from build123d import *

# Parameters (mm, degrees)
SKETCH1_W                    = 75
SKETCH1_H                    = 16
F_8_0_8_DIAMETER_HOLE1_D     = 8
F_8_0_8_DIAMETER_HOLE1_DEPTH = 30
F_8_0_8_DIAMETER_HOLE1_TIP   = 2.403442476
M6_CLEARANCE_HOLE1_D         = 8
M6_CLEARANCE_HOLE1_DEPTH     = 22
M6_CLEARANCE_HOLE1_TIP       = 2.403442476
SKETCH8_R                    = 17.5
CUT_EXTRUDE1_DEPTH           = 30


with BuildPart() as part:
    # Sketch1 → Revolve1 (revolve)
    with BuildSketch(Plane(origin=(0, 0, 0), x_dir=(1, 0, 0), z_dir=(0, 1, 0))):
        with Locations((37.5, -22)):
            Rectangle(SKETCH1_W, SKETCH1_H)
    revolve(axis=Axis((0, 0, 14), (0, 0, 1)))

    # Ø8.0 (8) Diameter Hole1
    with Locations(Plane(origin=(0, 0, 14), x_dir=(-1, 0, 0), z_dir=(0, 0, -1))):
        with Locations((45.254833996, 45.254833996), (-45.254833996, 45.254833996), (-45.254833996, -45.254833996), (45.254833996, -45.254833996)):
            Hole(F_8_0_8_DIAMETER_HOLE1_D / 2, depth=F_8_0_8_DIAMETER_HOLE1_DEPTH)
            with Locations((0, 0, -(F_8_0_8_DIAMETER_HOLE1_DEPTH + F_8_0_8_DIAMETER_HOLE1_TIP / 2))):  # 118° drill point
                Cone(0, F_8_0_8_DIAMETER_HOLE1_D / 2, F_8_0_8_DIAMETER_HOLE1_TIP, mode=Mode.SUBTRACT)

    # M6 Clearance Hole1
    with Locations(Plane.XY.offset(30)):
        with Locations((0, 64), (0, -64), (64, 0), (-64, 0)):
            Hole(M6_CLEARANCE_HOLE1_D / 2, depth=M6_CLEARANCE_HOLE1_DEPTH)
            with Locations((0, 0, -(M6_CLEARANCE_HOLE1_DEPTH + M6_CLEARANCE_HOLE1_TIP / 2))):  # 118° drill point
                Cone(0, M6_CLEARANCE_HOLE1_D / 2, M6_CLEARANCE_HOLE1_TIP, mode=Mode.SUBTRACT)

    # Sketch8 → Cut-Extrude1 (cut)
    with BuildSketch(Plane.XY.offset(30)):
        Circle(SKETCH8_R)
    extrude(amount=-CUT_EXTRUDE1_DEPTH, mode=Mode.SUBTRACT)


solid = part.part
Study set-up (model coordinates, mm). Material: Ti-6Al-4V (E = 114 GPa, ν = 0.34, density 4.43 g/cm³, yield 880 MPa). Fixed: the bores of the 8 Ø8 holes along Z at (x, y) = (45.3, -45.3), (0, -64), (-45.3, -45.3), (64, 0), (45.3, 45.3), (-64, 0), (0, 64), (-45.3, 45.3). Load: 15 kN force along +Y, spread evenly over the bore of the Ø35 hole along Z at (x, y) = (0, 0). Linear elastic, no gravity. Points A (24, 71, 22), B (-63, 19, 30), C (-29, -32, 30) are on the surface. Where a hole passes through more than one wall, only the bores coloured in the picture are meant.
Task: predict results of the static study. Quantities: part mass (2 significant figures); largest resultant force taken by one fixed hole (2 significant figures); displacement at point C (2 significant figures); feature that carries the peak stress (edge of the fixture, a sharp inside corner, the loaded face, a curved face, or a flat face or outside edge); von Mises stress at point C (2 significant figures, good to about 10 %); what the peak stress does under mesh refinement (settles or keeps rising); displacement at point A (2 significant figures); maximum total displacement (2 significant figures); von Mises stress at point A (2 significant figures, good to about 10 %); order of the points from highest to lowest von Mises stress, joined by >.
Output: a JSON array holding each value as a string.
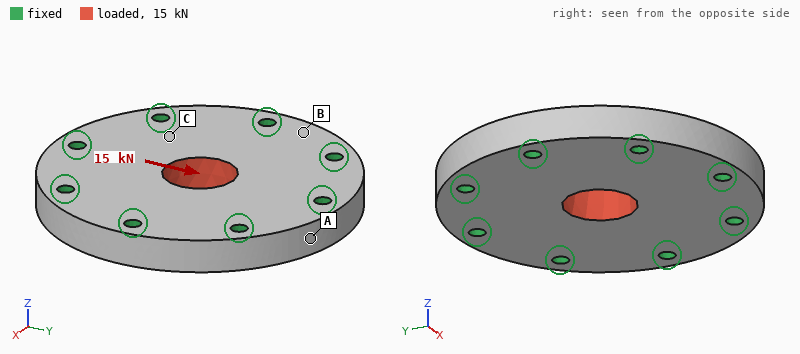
["1.2 kg", "3.1 kN", "1.2 µm", "edge of the fixture", "5.2 MPa", "keeps rising", "0.91 µm", "3.1 µm", "3.3 MPa", "C > A > B"]
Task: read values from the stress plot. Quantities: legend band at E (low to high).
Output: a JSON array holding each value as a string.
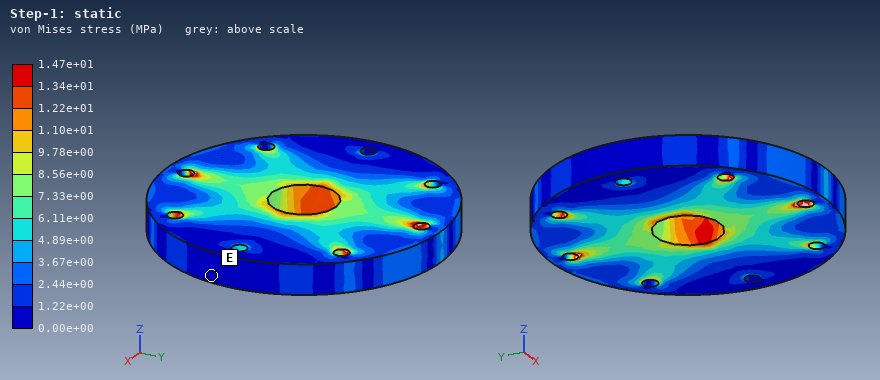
["0.00e+00 to 1.22e+00 MPa"]
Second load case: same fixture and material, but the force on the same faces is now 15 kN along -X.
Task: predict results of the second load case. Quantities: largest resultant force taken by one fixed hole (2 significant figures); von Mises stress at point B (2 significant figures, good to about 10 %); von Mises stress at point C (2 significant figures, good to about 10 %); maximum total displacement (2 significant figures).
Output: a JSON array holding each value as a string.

["3.1 kN", "1.7 MPa", "5.3 MPa", "3.1 µm"]
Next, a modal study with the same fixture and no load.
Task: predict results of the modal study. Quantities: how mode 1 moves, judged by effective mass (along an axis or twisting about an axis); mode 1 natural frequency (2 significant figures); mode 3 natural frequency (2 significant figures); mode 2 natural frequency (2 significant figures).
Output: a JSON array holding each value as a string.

["along Z", "7900 Hz", "13 kHz", "13 kHz"]
